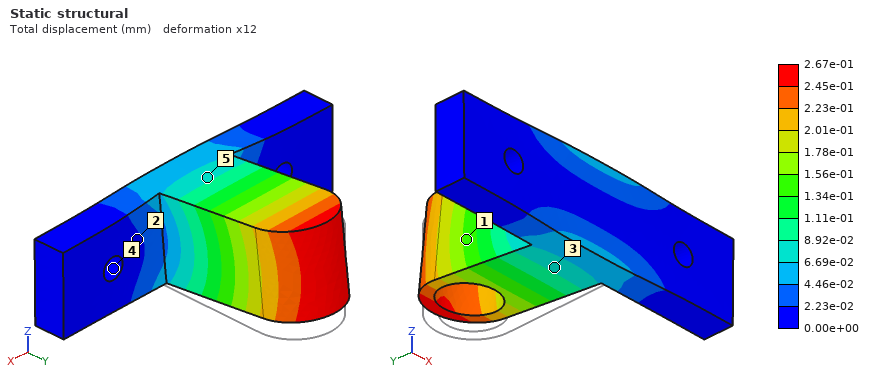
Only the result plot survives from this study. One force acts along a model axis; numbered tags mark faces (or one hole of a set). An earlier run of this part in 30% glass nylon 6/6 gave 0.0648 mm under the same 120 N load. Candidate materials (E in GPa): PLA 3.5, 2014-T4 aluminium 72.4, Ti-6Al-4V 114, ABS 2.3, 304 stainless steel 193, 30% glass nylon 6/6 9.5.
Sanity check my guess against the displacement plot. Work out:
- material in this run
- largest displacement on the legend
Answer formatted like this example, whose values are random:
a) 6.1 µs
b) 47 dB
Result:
a) ABS
b) 2.67e-01 mm
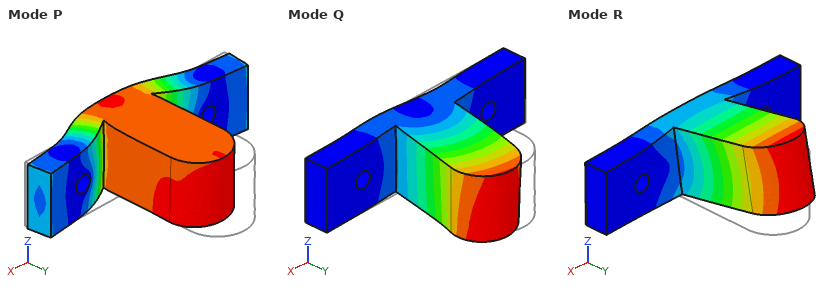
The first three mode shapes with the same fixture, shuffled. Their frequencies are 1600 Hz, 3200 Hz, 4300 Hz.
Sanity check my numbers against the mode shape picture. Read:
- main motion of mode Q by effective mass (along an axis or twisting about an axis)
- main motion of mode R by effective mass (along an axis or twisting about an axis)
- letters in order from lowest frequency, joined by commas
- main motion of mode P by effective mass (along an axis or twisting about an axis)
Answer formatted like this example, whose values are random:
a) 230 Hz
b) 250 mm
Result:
a) along X
b) along Z
c) R, Q, P
d) along Y
